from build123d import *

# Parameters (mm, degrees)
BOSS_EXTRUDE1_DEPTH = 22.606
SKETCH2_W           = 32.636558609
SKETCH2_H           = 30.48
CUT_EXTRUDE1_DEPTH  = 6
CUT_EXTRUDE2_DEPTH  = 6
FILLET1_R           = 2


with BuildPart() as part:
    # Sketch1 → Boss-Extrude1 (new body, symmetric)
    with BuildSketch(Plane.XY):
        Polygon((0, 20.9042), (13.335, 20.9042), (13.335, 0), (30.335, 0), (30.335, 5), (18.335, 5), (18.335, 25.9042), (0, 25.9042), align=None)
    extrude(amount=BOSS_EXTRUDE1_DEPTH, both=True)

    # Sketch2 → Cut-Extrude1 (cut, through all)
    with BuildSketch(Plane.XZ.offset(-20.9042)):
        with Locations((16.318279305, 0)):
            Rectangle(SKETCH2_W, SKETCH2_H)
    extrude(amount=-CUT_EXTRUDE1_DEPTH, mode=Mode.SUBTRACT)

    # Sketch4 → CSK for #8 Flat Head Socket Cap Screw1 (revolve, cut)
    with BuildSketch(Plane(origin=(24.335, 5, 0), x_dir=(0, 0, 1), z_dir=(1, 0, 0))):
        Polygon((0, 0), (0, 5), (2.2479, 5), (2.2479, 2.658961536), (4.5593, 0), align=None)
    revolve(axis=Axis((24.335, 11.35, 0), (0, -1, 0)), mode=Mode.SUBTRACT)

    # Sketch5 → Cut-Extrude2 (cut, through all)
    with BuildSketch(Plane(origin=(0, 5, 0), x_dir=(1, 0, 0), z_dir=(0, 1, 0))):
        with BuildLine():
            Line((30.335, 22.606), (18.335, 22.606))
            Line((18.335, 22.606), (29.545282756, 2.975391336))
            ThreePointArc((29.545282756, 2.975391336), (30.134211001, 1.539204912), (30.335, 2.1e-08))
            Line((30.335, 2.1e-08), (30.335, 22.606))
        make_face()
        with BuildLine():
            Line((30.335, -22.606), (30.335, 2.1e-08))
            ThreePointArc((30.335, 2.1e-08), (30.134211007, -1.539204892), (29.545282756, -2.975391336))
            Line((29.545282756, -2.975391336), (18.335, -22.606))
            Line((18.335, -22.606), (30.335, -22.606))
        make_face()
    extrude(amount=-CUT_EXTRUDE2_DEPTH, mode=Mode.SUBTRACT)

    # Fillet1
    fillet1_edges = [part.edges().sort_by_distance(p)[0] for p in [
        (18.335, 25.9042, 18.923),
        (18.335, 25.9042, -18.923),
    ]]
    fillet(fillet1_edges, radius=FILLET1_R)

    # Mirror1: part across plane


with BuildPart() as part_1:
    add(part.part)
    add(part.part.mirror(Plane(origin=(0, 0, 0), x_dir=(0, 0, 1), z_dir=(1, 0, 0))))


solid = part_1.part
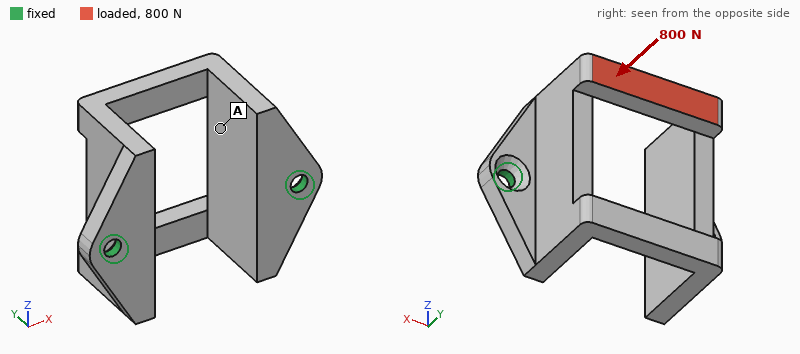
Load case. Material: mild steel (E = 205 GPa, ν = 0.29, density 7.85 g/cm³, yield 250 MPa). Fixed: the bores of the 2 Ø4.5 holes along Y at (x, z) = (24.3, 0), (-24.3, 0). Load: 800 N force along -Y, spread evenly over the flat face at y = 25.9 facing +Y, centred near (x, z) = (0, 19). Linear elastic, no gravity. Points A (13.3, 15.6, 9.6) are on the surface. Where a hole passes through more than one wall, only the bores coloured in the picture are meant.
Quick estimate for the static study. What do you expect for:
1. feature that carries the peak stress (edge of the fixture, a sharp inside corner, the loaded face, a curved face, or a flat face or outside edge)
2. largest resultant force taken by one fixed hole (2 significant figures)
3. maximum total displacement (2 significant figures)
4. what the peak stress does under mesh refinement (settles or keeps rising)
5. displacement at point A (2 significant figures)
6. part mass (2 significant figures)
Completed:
edge of the fixture
440 N
62 µm
keeps rising
29 µm
120 g
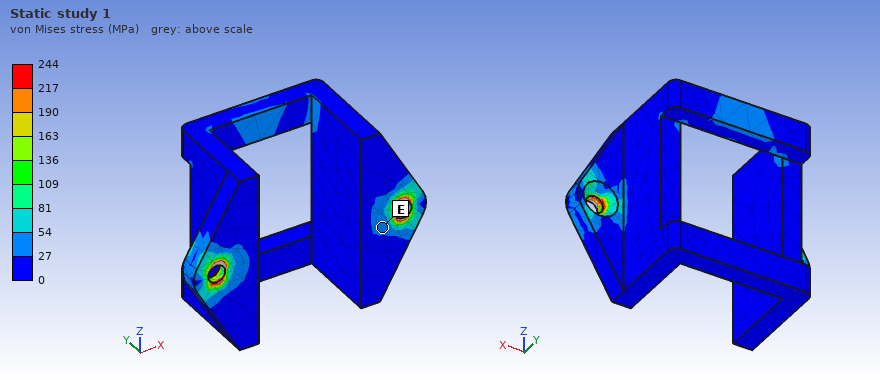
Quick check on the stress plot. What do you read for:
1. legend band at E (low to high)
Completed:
27 to 54 MPa
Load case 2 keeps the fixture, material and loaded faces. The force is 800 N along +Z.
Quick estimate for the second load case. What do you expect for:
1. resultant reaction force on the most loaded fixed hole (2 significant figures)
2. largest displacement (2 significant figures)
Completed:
400 N
84 µm
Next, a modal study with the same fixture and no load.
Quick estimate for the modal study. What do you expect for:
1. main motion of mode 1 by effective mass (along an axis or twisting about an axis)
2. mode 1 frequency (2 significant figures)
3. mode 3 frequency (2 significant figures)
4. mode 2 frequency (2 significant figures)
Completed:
along Z
2400 Hz
4800 Hz
4700 Hz
